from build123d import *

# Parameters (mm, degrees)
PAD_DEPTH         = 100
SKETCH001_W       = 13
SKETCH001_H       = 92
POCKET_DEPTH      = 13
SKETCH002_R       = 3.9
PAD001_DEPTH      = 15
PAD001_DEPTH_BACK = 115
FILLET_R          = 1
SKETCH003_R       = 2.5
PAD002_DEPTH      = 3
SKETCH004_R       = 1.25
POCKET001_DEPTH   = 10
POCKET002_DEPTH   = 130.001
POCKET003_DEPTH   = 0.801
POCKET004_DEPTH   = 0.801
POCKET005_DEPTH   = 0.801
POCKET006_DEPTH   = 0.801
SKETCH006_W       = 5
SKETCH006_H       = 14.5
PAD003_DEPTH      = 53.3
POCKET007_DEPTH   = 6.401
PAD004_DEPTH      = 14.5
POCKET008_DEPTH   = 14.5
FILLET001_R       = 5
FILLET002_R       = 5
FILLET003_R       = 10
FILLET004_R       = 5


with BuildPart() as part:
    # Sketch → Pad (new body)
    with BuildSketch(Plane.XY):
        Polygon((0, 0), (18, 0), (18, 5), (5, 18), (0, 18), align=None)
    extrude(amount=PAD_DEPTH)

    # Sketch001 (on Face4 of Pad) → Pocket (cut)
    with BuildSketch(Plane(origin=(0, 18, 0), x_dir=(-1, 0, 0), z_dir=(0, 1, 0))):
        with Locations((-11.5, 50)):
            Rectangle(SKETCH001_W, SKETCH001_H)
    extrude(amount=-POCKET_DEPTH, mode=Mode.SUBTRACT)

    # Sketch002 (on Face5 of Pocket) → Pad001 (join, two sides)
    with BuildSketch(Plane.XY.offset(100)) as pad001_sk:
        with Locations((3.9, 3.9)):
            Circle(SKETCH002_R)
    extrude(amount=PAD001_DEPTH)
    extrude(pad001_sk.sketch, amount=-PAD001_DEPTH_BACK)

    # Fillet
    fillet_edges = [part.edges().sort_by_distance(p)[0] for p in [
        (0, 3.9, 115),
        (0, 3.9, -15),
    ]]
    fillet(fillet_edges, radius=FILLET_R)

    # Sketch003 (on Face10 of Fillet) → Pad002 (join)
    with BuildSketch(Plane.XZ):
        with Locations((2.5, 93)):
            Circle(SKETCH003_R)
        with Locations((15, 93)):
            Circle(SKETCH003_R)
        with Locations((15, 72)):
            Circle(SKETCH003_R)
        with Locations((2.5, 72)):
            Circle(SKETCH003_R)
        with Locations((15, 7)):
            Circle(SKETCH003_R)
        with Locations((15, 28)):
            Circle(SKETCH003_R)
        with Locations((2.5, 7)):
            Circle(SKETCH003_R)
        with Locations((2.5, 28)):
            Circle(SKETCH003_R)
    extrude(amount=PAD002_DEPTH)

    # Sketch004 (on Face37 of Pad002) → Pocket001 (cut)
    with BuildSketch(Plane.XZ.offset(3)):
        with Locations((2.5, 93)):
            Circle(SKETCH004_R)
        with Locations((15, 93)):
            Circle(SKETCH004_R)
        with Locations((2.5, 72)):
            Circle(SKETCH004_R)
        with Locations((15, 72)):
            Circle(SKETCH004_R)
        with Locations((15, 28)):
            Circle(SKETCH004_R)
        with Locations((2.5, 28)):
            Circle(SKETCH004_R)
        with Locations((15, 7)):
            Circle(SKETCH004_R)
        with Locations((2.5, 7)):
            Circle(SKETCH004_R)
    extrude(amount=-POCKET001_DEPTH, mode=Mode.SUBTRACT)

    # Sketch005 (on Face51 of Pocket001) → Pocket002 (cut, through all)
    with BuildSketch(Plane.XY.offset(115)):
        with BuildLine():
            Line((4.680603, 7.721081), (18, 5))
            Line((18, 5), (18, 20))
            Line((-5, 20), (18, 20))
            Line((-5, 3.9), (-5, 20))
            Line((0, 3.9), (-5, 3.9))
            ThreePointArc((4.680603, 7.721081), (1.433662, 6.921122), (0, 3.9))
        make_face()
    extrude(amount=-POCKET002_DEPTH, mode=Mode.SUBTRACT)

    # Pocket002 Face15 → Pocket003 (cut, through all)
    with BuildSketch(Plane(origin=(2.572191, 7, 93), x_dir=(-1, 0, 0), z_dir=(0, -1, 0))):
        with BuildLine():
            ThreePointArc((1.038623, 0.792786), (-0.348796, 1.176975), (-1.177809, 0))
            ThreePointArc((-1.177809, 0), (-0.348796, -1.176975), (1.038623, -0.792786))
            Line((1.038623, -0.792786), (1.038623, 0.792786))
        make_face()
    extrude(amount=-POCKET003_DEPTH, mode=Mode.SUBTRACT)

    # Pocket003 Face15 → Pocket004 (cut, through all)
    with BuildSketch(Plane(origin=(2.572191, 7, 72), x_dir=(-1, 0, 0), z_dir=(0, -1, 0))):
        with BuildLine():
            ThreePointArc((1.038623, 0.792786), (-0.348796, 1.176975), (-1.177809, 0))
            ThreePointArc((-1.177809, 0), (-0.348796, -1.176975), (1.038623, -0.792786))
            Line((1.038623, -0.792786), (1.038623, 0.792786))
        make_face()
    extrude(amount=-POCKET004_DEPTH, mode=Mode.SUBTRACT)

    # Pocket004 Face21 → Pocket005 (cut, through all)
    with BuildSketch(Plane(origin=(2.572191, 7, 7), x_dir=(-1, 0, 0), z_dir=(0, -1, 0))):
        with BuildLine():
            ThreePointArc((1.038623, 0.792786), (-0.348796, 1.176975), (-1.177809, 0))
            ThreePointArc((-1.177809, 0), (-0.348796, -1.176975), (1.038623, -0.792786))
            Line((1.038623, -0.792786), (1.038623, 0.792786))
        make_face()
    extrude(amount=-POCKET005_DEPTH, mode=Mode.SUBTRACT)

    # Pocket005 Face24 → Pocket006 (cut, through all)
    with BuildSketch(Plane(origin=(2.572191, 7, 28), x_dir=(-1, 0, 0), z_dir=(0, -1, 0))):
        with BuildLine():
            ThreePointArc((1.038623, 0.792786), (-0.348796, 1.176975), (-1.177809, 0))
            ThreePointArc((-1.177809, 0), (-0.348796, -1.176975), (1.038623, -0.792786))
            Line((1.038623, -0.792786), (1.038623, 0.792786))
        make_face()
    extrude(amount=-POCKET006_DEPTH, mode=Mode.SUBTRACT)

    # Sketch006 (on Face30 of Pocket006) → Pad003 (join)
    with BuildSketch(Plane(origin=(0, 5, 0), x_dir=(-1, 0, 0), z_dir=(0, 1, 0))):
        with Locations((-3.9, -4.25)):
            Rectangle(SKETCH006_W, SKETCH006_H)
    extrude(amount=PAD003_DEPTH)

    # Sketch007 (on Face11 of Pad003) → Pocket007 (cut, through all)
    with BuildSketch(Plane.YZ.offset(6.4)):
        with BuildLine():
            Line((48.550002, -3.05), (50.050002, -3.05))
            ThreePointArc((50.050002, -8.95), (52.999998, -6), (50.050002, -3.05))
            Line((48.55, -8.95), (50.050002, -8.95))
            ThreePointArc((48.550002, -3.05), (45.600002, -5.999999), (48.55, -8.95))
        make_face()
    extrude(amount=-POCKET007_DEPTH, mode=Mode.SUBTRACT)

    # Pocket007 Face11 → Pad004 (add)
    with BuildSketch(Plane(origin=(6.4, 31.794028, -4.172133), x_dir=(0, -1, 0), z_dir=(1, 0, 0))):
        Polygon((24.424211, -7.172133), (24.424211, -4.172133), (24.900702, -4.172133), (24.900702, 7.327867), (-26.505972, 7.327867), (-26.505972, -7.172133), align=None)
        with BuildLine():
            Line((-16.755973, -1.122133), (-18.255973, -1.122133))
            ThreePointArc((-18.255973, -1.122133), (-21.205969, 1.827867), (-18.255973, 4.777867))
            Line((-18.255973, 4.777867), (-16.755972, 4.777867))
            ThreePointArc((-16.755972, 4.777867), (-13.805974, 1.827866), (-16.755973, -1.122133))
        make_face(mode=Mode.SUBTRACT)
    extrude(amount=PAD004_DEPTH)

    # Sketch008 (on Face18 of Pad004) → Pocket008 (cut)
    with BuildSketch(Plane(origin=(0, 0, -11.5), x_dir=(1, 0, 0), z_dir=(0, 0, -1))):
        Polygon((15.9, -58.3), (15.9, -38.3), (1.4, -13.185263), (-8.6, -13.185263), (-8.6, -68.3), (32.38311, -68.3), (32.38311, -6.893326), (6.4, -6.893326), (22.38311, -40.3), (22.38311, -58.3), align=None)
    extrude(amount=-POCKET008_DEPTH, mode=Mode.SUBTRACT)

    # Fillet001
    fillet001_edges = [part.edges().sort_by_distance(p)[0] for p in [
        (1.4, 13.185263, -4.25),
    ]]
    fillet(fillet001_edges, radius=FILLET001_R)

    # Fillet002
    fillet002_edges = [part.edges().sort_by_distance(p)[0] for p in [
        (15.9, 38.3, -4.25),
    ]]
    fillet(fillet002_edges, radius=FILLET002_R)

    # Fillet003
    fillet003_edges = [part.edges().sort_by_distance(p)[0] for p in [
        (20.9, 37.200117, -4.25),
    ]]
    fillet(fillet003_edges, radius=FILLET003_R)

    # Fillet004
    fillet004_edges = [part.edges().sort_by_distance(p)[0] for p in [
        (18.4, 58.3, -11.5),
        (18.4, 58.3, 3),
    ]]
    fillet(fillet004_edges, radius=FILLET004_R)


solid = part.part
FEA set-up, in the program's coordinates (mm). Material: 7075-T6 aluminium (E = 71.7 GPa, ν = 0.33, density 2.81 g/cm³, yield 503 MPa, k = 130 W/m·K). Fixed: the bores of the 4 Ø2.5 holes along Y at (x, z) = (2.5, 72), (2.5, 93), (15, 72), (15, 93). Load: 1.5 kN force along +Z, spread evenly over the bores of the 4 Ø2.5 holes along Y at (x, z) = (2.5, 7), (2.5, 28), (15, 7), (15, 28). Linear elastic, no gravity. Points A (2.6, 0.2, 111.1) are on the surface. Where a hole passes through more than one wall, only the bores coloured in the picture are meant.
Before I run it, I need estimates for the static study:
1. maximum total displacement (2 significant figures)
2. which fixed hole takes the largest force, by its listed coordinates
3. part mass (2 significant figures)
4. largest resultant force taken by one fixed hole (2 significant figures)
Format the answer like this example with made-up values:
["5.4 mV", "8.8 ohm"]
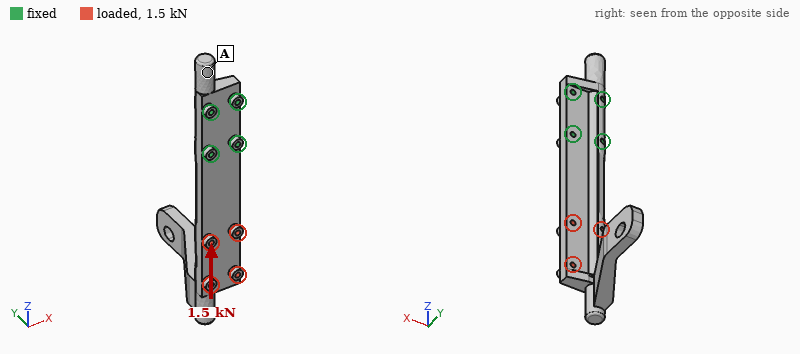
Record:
["0.37 mm", "(2.5, 72)", "46 g", "800 N"]
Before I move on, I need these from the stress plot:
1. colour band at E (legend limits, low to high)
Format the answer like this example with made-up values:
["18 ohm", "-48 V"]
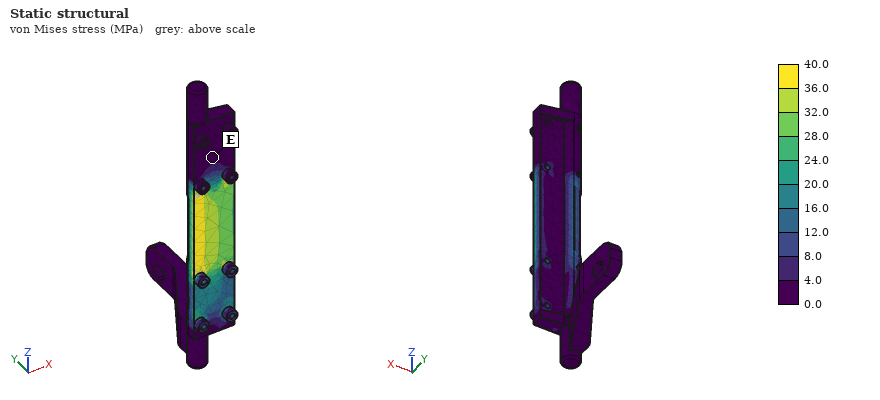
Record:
["0.0 to 4.0 MPa"]
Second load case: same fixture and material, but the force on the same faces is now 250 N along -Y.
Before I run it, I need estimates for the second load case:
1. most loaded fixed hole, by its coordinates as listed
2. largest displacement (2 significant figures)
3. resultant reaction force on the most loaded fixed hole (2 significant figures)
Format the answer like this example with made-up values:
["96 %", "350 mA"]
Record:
["(2.5, 72)", "1.3 mm", "280 N"]
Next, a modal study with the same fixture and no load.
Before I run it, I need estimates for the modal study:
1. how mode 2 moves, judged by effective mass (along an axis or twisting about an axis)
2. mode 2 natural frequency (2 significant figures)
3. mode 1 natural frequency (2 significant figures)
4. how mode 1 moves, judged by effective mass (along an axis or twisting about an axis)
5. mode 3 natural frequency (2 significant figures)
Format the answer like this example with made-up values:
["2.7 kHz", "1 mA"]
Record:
["along X", "720 Hz", "430 Hz", "along Y", "1600 Hz"]
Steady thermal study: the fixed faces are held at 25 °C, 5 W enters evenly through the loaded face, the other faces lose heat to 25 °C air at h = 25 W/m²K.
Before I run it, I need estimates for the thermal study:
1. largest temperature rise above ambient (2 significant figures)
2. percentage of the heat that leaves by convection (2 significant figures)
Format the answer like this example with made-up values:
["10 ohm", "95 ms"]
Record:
["14 K", "31 %"]
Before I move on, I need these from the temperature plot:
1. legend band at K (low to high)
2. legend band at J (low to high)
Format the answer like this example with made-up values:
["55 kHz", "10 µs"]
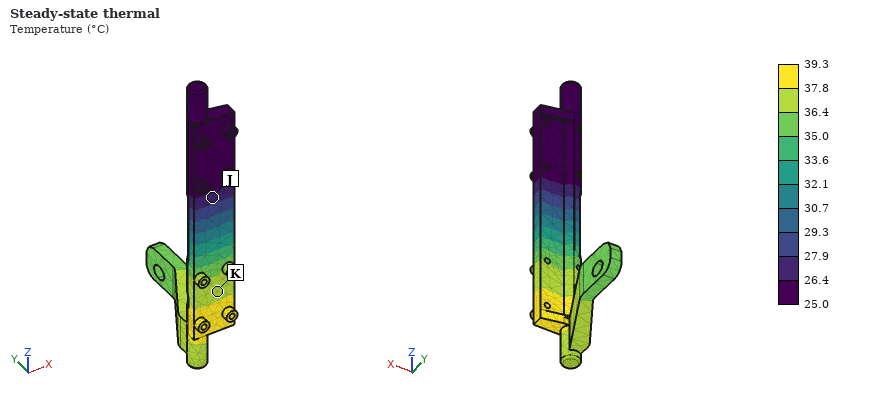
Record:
["36.4 to 37.8 °C", "26.4 to 27.9 °C"]
